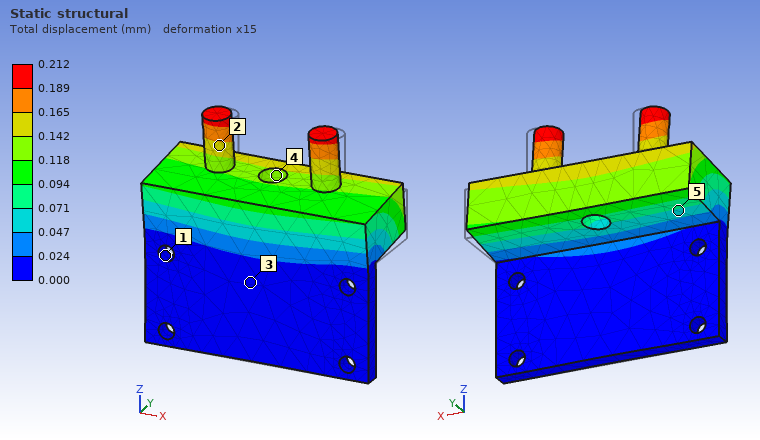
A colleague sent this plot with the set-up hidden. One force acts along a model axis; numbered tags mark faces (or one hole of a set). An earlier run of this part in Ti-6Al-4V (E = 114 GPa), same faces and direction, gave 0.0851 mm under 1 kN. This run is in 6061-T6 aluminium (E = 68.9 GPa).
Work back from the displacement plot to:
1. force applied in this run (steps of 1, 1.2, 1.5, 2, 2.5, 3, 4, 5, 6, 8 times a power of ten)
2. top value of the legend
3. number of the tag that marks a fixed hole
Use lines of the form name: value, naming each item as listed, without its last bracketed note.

force applied in this run: 1.5 kN
top value of the legend: 0.212 mm
number of the tag that marks a fixed hole: 1
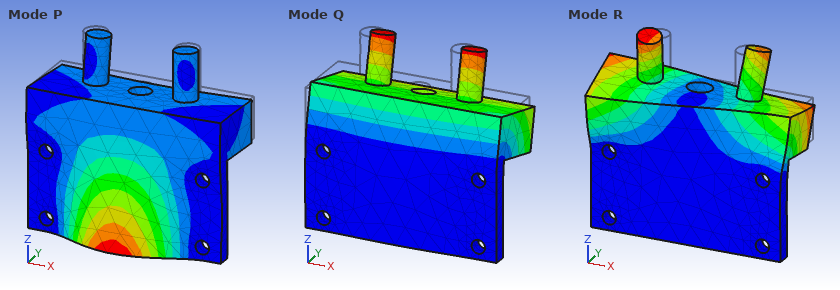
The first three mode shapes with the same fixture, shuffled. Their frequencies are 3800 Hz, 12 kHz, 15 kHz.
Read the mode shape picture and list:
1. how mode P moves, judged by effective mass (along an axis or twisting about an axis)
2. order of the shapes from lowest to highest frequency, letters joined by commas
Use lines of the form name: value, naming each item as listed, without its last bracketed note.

how mode P moves, judged by effective mass: along Y
order of the shapes from lowest to highest frequency, letters joined by commas: Q, R, P
